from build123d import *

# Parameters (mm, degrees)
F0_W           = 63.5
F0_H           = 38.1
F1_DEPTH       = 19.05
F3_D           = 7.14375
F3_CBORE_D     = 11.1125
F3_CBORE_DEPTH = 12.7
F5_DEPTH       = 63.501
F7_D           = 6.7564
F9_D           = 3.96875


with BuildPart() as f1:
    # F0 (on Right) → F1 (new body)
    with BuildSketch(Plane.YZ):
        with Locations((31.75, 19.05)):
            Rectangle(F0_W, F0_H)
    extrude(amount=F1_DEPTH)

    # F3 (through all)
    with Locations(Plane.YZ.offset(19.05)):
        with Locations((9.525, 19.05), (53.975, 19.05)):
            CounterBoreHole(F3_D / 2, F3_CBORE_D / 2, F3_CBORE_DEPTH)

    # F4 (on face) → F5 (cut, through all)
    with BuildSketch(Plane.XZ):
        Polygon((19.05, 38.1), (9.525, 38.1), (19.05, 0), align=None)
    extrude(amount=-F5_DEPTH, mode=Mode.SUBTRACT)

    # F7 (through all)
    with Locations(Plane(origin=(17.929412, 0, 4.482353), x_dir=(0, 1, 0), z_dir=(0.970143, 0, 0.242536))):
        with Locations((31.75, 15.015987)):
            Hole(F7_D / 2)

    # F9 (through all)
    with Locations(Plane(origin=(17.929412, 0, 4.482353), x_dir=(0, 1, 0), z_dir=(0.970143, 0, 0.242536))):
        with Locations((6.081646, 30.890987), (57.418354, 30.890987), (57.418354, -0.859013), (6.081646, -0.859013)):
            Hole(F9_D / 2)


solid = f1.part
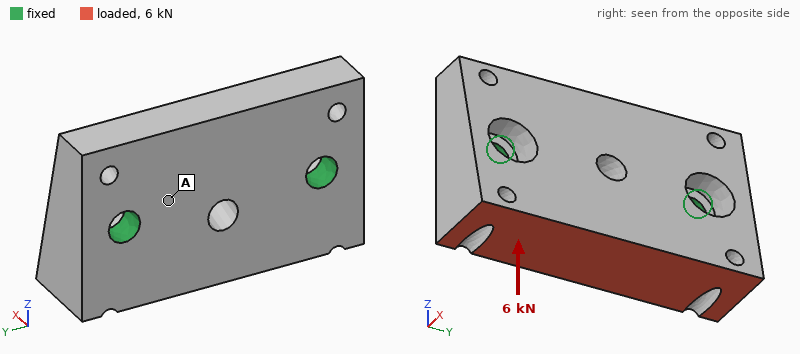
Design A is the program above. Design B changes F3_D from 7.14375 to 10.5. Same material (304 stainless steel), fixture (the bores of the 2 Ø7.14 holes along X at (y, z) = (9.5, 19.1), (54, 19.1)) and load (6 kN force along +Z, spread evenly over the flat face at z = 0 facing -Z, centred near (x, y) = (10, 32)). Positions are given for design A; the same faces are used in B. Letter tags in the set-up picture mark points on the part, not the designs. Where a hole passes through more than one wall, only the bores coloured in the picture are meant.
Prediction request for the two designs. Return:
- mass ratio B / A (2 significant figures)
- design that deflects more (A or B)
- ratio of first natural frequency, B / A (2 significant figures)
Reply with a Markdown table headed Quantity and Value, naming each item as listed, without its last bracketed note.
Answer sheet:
| Quantity | Value |
|---|---|
| mass ratio B / A | 0.98 |
| design that deflects more | A |
| ratio of first natural frequency, B / A | 1.4 |
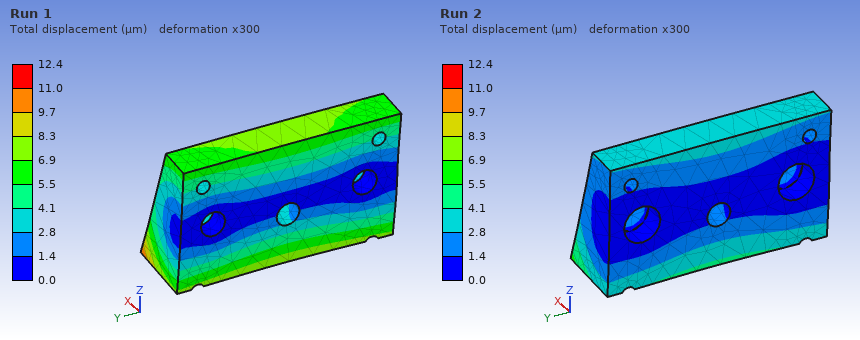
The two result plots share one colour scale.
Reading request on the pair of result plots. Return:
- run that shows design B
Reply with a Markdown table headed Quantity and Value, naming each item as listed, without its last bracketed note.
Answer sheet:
| Quantity | Value |
|---|---|
| run that shows design B | Run 2 |
